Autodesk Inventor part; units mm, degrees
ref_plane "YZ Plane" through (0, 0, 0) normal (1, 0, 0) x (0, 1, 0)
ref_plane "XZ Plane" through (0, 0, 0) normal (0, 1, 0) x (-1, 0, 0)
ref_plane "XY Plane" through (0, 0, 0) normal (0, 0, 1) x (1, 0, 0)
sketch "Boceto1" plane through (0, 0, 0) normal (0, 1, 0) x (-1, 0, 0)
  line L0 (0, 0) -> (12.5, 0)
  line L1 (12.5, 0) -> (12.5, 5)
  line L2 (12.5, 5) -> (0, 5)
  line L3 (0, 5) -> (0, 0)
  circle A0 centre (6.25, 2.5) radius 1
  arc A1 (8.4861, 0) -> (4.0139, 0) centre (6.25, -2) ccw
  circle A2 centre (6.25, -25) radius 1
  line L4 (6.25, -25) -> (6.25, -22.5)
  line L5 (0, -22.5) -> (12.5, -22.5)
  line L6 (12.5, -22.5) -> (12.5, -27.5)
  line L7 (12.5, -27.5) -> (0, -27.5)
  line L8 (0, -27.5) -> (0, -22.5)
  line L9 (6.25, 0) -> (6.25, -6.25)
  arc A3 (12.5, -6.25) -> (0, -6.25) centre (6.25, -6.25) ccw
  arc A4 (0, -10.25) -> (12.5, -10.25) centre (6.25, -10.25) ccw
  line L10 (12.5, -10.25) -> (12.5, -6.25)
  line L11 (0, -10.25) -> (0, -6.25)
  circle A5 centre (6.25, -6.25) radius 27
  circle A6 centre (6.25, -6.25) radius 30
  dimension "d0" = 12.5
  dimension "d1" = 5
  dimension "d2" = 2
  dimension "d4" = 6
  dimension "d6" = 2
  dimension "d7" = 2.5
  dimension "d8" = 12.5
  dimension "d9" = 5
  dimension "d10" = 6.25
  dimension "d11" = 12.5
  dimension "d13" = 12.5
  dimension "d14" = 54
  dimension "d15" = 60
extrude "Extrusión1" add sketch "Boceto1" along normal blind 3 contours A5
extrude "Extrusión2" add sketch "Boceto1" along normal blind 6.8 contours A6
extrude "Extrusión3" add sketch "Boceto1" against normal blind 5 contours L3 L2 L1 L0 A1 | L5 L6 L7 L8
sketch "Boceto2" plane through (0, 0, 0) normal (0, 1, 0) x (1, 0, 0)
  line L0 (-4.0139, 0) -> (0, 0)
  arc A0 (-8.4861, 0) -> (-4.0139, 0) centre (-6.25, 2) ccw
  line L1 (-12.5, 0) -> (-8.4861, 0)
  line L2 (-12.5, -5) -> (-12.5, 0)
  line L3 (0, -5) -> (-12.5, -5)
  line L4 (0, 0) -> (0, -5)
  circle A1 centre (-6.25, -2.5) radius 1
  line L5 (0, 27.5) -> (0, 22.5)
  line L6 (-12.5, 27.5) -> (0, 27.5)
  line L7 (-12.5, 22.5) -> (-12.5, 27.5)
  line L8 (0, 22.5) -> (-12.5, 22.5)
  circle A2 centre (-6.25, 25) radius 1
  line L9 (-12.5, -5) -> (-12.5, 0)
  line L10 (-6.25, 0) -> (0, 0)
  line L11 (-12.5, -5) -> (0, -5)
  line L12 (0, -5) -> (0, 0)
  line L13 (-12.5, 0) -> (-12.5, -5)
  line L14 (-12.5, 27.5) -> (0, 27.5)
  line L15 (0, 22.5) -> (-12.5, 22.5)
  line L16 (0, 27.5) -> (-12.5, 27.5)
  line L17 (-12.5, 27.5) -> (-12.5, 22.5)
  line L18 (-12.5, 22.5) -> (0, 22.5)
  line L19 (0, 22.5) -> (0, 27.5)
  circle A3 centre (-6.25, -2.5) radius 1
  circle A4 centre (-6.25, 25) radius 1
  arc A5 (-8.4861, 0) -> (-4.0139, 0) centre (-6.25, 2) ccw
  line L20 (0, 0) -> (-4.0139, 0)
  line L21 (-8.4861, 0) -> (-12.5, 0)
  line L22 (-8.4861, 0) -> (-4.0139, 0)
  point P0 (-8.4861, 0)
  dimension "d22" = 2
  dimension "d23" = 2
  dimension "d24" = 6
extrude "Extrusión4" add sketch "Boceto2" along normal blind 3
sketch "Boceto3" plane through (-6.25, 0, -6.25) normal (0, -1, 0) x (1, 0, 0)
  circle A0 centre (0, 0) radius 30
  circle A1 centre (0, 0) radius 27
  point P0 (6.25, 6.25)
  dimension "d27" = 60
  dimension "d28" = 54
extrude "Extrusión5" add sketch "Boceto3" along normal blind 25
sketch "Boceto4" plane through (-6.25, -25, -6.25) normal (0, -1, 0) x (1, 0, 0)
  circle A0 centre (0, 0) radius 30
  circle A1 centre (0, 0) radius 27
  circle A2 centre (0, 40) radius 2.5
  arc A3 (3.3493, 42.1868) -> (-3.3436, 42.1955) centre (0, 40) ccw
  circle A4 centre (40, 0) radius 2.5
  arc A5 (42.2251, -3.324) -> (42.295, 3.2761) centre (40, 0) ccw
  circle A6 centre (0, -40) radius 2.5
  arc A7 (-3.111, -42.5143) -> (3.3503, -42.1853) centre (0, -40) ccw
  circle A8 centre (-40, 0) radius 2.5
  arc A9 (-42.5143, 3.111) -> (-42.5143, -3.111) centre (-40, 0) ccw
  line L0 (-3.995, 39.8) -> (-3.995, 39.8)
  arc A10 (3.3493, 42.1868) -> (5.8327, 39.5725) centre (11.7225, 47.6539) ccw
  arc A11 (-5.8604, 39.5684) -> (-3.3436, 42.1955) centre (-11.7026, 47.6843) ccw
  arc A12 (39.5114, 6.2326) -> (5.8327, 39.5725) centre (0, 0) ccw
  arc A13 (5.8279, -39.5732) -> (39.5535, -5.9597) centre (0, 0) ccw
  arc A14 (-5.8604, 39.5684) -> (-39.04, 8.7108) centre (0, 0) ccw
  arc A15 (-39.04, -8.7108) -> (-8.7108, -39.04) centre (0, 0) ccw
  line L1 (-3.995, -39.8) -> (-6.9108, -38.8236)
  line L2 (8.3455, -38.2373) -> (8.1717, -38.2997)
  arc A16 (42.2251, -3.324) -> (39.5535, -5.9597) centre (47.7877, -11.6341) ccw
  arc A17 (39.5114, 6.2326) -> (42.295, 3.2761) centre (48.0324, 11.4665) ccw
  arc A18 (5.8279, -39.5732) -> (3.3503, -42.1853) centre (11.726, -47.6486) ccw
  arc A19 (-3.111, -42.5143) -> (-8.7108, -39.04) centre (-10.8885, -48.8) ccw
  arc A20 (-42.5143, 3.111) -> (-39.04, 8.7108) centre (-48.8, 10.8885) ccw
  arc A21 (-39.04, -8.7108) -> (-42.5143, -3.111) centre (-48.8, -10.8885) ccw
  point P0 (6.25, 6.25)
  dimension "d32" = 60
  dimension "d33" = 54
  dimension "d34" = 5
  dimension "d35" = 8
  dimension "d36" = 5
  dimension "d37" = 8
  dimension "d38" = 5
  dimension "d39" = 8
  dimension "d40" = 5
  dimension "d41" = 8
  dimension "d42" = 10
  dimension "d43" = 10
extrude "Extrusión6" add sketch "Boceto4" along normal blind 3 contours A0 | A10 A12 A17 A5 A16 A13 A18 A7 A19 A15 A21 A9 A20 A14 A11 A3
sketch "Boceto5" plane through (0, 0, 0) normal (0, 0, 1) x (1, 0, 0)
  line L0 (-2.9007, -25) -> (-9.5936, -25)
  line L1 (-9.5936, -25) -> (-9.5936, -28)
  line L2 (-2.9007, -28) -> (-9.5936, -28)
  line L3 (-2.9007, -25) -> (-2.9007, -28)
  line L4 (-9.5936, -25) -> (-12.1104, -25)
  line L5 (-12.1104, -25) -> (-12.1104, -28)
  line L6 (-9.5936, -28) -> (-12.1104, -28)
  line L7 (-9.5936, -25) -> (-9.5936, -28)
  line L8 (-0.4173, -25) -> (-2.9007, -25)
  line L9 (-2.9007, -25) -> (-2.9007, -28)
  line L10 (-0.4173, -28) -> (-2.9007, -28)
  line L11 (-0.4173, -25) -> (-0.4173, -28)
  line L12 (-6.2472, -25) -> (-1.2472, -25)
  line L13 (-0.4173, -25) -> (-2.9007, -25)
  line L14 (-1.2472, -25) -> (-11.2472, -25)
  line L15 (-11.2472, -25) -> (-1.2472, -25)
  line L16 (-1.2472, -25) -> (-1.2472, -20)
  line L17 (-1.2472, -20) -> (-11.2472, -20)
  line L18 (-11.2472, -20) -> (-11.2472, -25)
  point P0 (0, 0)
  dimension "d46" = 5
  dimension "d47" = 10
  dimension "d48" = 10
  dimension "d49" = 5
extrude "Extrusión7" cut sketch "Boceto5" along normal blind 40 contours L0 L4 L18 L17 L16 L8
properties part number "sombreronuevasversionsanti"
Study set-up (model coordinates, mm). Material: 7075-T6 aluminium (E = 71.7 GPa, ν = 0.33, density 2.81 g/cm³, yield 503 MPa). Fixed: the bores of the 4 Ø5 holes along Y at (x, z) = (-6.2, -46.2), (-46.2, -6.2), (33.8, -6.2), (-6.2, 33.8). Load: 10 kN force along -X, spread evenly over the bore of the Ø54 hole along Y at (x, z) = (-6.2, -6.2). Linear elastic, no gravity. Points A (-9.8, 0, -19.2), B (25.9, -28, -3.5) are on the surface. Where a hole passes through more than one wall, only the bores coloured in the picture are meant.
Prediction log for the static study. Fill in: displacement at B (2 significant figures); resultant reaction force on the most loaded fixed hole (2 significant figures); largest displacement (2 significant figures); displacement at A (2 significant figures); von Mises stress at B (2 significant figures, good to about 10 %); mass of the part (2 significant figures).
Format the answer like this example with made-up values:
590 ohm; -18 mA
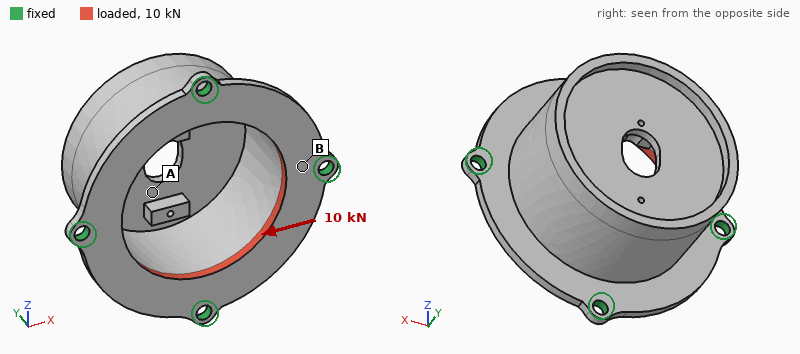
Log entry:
5.7 µm; 2.8 kN; 33 µm; 17 µm; 55 MPa; 90 g
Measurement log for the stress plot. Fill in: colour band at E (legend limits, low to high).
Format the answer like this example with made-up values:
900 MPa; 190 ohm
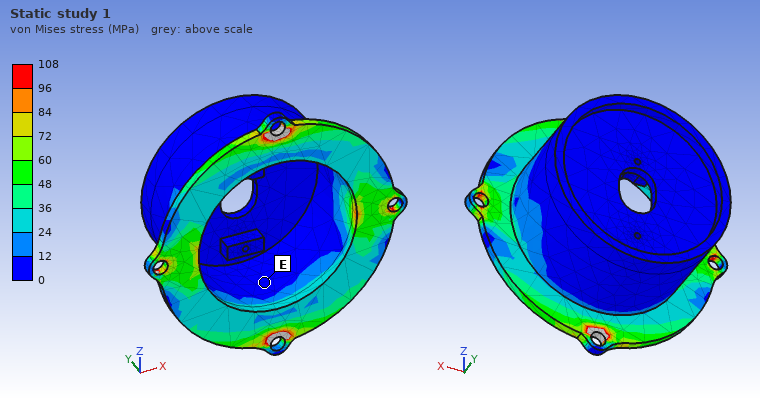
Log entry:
0 to 12 MPa
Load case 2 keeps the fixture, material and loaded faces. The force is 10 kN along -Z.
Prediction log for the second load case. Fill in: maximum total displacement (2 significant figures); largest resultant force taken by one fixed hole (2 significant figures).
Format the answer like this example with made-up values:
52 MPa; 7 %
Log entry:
34 µm; 2.8 kN
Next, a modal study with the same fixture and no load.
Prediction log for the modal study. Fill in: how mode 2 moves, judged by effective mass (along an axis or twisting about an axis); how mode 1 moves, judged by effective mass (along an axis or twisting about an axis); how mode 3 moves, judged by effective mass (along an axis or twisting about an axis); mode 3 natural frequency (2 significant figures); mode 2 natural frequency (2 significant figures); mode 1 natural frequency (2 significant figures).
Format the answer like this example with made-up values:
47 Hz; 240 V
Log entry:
along X; along Z; along Y; 4400 Hz; 3900 Hz; 3600 Hz
